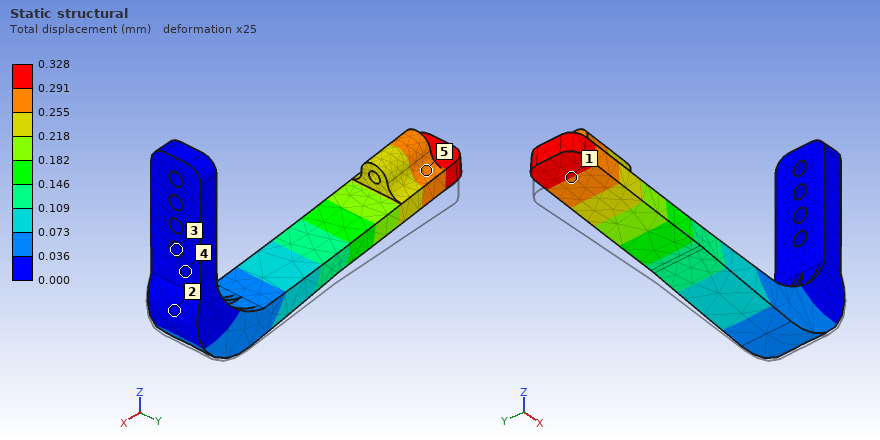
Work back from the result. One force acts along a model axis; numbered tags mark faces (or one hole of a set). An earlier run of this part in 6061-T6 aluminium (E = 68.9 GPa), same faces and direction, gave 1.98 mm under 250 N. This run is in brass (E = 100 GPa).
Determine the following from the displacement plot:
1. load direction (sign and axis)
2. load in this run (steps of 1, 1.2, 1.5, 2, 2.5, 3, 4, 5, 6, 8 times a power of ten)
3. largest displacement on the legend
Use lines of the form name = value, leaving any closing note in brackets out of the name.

load direction = +Z
load in this run = 60 N
largest displacement on the legend = 0.328 mm
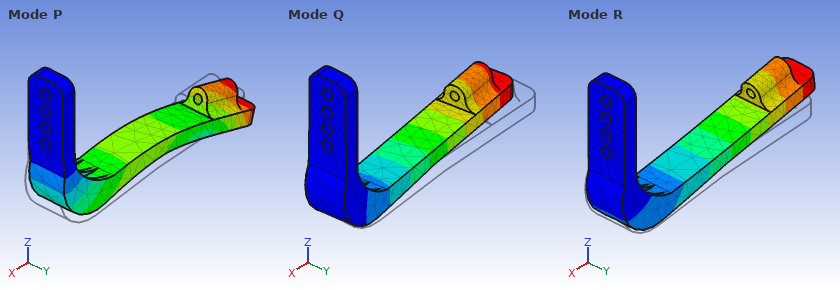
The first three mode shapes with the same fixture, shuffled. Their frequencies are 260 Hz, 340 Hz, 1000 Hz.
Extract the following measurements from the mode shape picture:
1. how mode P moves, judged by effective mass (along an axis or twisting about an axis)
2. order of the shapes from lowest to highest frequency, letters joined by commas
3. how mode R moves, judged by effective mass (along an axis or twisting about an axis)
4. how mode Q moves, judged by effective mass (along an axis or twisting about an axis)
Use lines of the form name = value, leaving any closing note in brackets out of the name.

how mode P moves, judged by effective mass = along X
order of the shapes from lowest to highest frequency, letters joined by commas = R, Q, P
how mode R moves, judged by effective mass = along Z
how mode Q moves, judged by effective mass = along Y
